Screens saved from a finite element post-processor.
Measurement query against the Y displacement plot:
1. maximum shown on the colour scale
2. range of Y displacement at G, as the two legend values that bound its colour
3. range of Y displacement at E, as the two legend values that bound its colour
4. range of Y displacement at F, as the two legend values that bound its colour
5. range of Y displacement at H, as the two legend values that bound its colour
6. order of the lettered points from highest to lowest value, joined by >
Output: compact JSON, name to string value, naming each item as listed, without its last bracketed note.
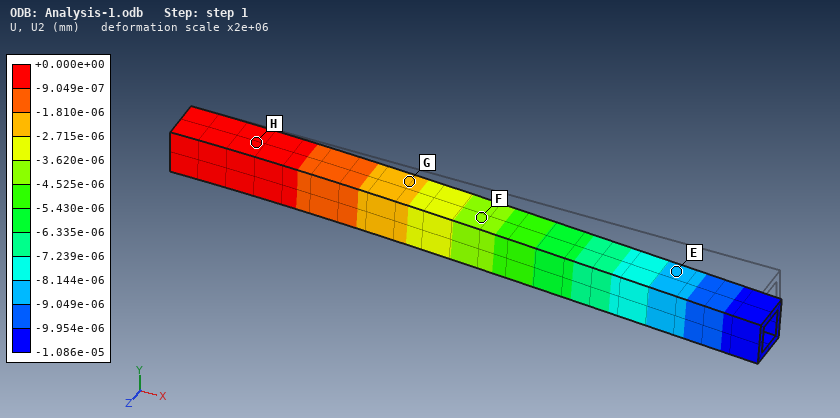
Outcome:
{"maximum shown on the colour scale": "+0.000e+00 mm", "range of Y displacement at G, as the two legend values that bound its colour": "-2.715e-06 to -1.810e-06 mm", "range of Y displacement at E, as the two legend values that bound its colour": "-9.049e-06 to -8.144e-06 mm", "range of Y displacement at F, as the two legend values that bound its colour": "-4.525e-06 to -3.620e-06 mm", "range of Y displacement at H, as the two legend values that bound its colour": "-9.049e-07 to +0.000e+00 mm", "order of the lettered points from highest to lowest value, joined by >": "H > G > F > E"}
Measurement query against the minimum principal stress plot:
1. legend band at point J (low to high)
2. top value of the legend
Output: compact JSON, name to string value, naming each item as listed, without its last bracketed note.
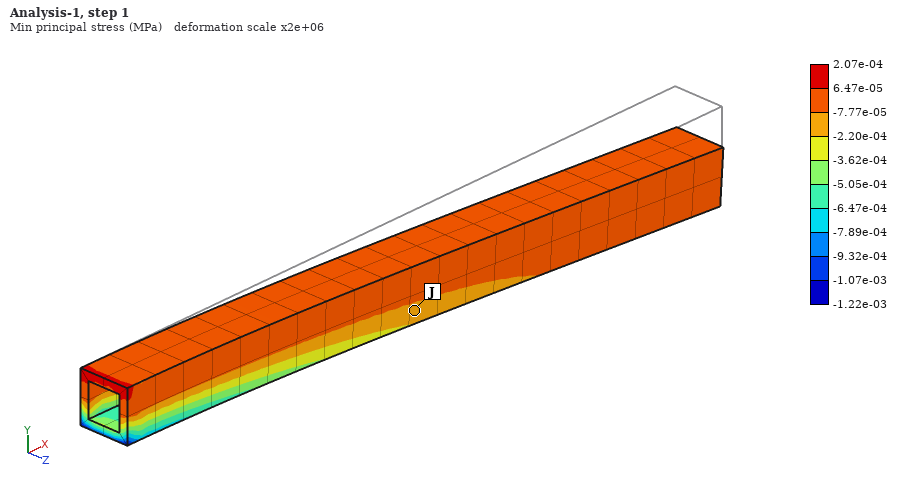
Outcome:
{"legend band at point J": "-2.20e-04 to -7.77e-05 MPa", "top value of the legend": "2.07e-04 MPa"}
